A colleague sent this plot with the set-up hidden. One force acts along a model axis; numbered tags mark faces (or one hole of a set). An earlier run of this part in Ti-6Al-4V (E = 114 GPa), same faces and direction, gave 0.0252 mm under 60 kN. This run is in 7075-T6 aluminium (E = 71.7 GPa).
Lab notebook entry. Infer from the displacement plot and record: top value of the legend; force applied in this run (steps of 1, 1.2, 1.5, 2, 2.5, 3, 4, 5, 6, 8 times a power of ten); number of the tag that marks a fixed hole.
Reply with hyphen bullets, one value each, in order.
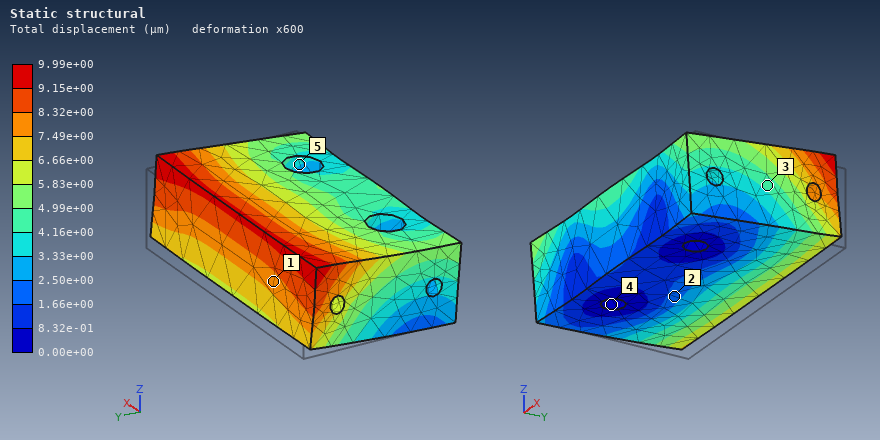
- 9.99e+00 µm
- 15 kN
- 4
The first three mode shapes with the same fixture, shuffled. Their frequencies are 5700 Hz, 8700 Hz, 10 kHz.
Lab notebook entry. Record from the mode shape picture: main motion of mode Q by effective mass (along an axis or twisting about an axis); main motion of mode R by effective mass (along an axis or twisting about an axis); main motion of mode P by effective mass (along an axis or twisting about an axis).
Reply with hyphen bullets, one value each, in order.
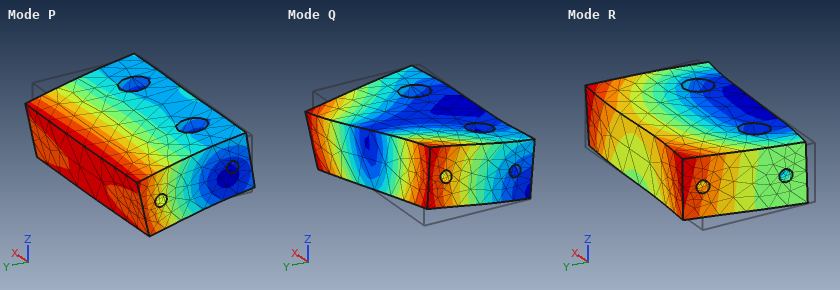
- twisting about Y
- along X
- along Z
